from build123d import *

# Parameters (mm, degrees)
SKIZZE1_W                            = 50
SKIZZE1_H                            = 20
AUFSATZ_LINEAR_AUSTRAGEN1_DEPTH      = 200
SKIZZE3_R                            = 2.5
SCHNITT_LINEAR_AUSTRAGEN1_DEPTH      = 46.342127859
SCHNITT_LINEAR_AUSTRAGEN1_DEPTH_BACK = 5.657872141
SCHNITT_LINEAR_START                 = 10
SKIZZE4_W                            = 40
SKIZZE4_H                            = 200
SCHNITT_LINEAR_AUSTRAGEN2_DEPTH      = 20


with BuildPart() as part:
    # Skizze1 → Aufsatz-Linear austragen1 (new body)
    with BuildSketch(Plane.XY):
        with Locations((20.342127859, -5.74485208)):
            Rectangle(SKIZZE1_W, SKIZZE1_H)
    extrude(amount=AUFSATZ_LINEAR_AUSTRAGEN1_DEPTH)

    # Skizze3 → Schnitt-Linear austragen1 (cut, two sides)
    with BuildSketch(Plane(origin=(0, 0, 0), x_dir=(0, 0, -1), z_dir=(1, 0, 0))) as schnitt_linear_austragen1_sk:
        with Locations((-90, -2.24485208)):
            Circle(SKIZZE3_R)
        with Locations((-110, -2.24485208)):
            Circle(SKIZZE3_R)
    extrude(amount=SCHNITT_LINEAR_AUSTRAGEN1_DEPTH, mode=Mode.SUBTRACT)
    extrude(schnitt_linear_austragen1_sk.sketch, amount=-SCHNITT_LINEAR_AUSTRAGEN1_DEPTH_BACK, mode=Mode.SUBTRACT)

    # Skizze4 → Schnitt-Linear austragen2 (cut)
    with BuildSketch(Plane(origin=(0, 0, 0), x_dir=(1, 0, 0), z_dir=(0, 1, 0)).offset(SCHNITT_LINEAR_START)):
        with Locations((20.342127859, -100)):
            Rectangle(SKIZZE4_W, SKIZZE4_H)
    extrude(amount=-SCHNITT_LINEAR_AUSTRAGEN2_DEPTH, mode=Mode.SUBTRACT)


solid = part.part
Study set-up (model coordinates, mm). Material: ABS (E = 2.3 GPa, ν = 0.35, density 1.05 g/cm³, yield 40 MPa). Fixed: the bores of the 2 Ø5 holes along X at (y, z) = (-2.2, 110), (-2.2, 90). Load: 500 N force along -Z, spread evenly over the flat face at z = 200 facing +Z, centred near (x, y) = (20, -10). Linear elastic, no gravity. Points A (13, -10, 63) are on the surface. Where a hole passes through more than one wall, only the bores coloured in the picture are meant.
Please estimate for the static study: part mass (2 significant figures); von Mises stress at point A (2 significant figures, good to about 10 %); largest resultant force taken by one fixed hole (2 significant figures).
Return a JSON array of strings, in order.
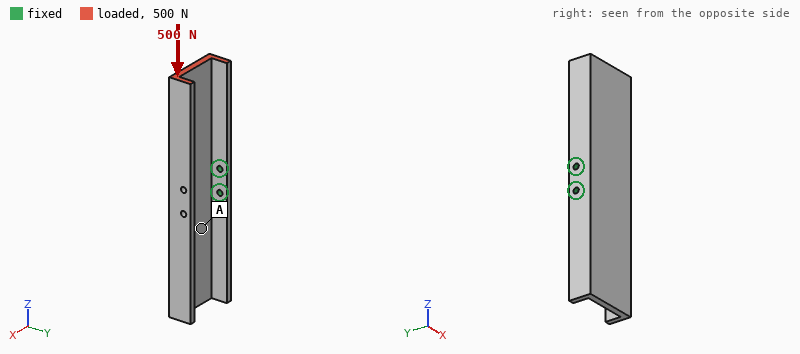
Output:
["90 g", "2.3 MPa", "530 N"]
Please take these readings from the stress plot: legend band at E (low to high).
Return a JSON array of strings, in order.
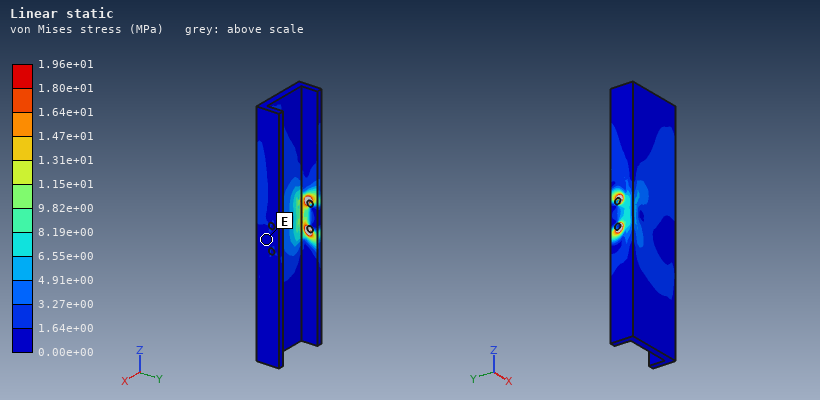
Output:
["0.00e+00 to 1.64e+00 MPa"]
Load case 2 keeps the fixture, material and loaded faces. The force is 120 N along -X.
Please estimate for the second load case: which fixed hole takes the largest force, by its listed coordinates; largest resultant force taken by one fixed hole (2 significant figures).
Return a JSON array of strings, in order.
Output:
["(-2.2, 110)", "500 N"]
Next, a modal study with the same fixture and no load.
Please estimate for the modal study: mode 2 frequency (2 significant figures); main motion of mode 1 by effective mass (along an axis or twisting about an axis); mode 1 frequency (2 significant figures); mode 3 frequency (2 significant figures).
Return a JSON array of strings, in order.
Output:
["180 Hz", "along Y", "180 Hz", "240 Hz"]
